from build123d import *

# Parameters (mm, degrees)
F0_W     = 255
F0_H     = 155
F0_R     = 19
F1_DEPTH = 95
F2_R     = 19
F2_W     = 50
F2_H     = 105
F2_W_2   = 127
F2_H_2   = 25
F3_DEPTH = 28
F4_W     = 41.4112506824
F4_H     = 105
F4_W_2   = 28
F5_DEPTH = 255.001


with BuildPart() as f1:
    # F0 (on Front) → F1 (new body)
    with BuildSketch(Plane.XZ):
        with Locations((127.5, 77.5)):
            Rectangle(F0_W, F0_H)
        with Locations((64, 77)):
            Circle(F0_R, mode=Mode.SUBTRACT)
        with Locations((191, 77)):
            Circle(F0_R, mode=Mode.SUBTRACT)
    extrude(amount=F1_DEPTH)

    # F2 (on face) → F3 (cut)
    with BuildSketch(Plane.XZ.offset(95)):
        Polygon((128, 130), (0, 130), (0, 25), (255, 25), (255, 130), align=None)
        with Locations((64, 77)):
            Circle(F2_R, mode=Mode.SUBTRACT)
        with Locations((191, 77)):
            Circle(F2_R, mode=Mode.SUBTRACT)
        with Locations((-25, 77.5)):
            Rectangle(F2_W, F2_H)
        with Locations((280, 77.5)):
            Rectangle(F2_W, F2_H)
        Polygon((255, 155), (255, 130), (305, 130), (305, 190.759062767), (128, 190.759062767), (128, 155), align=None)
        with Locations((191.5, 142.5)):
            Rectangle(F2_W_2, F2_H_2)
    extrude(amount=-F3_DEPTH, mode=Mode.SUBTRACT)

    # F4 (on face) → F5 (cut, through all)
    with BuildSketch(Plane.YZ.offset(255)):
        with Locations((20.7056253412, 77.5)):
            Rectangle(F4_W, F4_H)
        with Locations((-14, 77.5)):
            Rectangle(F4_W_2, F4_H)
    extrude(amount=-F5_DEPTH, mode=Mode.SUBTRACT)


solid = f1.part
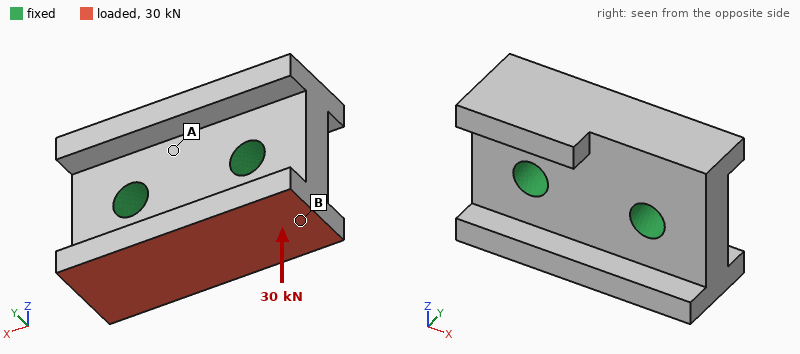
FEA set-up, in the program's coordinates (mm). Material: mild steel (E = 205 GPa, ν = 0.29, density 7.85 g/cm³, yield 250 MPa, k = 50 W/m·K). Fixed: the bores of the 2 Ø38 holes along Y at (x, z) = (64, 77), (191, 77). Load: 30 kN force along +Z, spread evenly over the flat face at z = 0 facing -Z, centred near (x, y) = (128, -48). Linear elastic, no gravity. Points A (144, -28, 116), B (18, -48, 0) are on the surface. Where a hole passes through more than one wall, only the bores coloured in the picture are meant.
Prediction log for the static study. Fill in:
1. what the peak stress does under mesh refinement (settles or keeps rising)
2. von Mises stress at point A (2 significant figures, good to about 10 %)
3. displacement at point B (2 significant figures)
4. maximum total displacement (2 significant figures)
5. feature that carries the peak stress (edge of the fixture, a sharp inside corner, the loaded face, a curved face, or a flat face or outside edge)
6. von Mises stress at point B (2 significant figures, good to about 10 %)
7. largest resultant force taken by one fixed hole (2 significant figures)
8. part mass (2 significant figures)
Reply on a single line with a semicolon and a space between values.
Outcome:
keeps rising; 0.77 MPa; 1.2 µm; 2.8 µm; edge of the fixture; 4.9 MPa; 15 kN; 16 kg
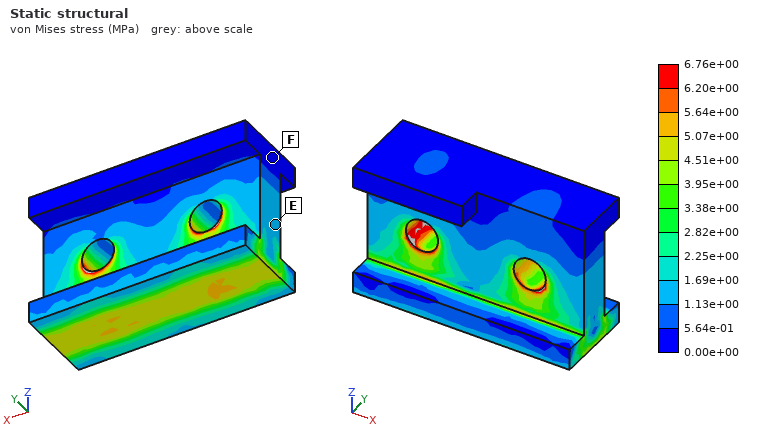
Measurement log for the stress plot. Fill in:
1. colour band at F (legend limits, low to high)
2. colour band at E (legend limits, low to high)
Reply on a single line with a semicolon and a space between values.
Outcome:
0.00e+00 to 5.64e-01 MPa; 1.13e+00 to 1.69e+00 MPa
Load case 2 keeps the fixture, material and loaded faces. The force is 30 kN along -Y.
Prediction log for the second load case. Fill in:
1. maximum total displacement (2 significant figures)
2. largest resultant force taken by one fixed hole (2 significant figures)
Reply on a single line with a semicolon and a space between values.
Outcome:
23 µm; 15 kN
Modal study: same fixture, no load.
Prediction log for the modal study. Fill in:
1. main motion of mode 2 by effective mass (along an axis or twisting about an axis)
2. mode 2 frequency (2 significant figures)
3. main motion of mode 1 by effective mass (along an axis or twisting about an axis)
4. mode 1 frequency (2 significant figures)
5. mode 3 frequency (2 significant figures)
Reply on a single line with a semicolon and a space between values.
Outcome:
along Y; 3500 Hz; twisting about X; 3100 Hz; 3700 Hz
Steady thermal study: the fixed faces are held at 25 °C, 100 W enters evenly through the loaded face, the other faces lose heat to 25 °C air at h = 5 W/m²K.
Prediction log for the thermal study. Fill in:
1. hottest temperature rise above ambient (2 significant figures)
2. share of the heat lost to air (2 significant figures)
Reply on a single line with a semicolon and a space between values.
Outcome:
14 K; 3.2 %
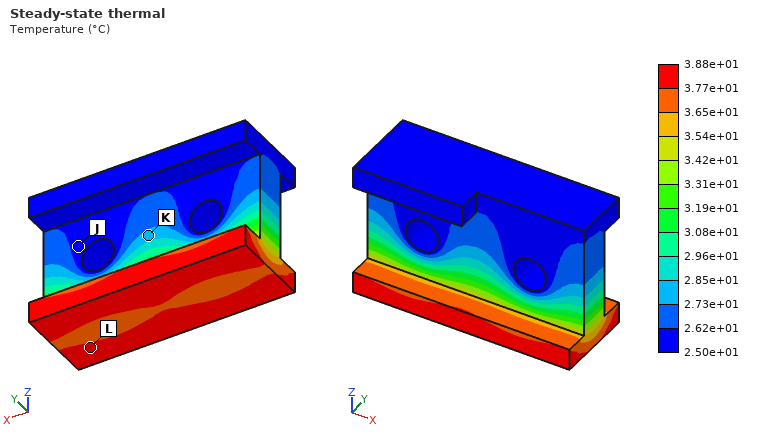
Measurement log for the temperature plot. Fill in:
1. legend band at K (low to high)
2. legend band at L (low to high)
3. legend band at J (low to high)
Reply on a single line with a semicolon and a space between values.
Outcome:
2.73e+01 to 2.85e+01 °C; 3.77e+01 to 3.88e+01 °C; 2.50e+01 to 2.62e+01 °C
